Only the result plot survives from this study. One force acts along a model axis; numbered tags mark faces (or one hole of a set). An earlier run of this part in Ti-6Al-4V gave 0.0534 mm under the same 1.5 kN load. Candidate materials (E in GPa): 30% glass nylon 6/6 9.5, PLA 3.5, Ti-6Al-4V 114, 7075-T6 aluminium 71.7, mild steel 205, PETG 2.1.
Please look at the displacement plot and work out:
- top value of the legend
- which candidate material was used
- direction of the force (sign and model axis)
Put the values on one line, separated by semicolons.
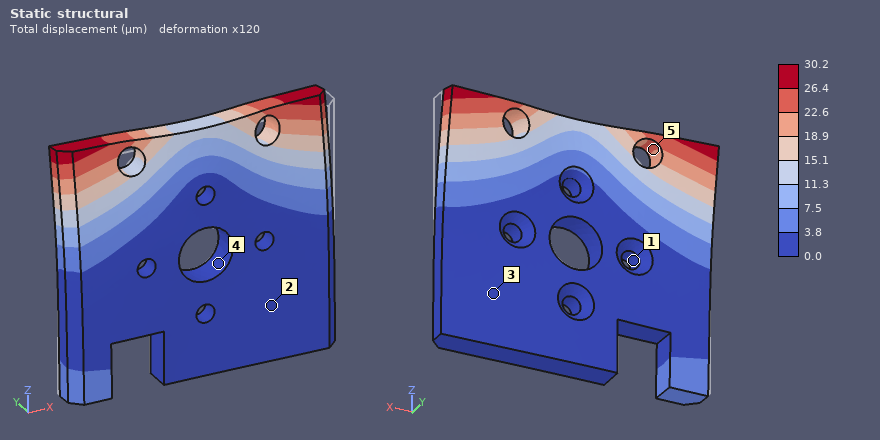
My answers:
30.2 µm; mild steel; +Y
